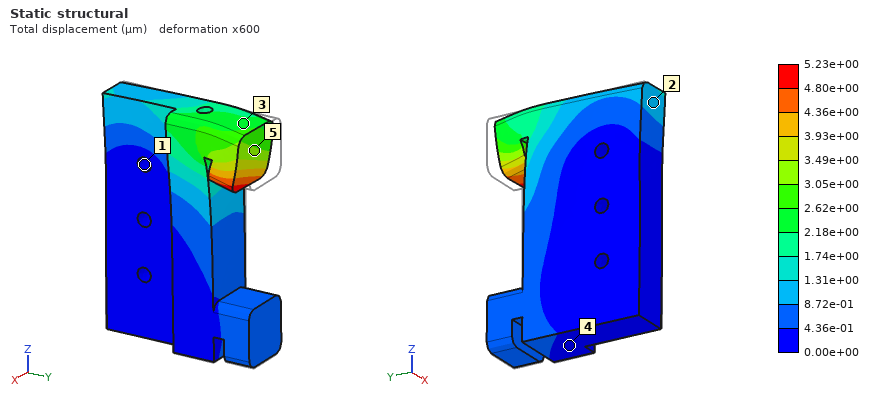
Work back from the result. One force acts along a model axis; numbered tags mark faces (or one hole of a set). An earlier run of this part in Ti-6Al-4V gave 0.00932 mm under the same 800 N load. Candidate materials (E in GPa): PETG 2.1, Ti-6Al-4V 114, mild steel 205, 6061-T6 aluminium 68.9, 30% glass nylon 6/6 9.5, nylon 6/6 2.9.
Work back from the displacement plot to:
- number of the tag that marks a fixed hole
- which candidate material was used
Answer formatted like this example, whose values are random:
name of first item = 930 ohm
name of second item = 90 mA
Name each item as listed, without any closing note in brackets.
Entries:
number of the tag that marks a fixed hole = 1
which candidate material was used = mild steel
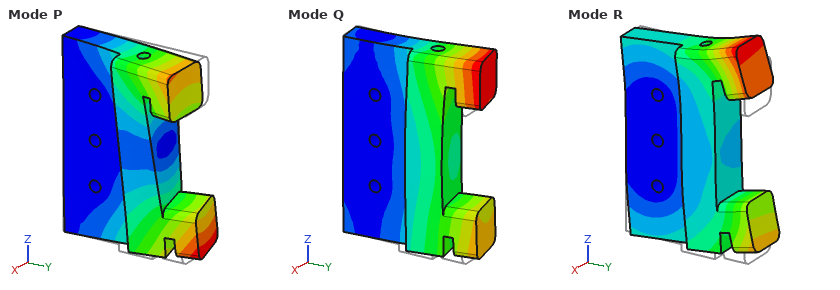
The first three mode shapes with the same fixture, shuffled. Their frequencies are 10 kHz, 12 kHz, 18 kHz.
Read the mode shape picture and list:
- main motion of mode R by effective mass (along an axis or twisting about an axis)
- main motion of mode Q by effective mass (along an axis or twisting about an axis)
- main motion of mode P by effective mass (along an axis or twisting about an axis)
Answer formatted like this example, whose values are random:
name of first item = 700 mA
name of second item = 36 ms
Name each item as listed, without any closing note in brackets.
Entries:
main motion of mode R by effective mass = along Z
main motion of mode Q by effective mass = along X
main motion of mode P by effective mass = twisting about Y
